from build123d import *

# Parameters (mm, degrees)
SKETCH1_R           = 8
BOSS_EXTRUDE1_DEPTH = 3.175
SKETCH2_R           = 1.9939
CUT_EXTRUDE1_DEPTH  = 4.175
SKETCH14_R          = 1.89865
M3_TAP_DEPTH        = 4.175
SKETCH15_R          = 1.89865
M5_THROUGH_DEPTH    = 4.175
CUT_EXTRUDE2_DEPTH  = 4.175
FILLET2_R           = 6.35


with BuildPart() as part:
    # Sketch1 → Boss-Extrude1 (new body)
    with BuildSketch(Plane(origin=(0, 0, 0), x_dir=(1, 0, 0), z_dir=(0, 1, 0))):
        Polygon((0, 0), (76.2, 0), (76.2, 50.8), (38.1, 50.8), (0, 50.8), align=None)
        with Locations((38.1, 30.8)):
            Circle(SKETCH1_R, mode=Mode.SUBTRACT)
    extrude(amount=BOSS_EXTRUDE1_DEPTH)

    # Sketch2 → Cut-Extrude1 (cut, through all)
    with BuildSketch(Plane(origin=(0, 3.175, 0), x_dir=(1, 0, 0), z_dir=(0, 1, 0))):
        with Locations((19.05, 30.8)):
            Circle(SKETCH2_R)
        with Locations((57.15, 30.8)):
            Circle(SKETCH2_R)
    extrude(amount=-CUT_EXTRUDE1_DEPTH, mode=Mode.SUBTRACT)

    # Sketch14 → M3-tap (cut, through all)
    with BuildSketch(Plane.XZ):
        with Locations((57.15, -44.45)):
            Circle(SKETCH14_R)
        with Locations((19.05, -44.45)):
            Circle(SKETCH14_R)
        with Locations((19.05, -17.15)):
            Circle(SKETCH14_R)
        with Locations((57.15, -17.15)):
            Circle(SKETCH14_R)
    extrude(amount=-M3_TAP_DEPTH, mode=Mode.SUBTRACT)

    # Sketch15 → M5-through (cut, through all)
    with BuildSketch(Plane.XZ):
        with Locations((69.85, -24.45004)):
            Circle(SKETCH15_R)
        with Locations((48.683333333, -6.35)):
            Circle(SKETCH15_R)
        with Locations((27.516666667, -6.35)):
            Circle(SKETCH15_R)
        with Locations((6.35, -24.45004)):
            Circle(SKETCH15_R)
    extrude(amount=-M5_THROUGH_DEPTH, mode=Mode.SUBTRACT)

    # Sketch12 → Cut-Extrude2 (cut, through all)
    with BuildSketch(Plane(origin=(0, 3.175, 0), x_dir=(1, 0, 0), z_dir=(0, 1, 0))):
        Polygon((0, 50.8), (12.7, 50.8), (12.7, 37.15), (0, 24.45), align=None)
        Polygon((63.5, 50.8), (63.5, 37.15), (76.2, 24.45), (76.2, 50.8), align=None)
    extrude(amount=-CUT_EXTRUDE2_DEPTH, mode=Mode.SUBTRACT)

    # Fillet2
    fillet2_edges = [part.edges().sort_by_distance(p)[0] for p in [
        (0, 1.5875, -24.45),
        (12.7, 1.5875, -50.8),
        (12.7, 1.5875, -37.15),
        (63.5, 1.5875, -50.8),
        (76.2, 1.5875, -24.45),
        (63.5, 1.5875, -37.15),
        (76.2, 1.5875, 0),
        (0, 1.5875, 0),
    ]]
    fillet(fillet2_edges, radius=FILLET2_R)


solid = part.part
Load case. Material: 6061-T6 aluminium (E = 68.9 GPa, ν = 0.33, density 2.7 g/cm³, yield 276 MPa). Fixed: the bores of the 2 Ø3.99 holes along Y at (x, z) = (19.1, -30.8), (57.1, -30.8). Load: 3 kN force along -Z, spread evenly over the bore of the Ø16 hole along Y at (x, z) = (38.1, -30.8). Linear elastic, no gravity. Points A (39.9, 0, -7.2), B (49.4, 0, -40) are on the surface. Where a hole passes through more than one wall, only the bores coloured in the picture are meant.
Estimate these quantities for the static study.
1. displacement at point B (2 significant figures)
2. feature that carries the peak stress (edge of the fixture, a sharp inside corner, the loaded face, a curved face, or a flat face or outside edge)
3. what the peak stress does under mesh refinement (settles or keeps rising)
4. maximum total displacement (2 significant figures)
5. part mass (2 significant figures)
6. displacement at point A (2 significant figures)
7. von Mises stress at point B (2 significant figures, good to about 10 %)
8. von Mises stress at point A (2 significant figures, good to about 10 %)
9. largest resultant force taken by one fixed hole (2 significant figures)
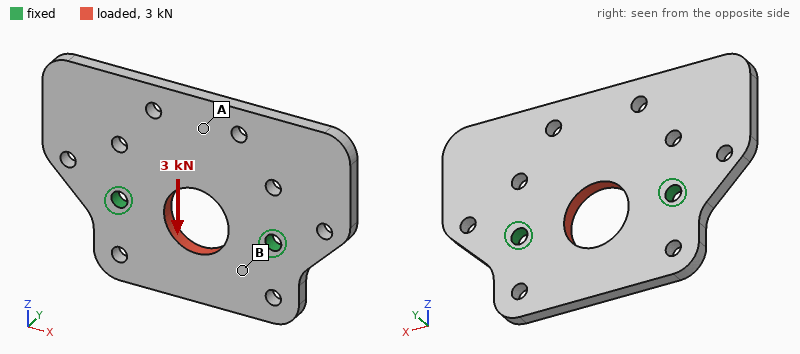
6.5 µm
edge of the fixture
keeps rising
12 µm
26 g
7.1 µm
22 MPa
8.6 MPa
1.5 kN
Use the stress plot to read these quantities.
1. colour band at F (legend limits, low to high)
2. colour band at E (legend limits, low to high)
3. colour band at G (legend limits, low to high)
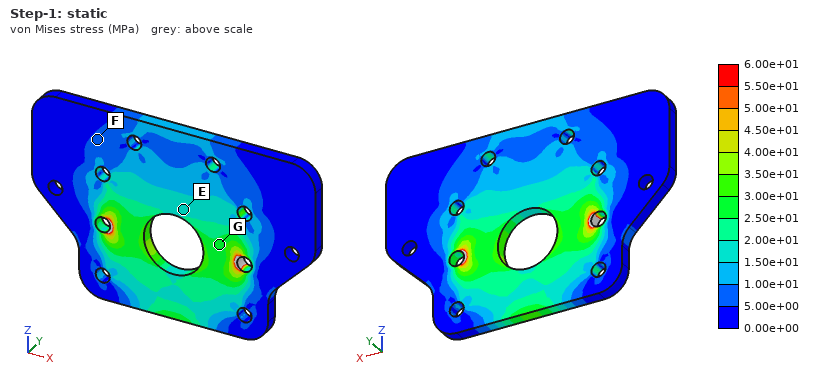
5.00e+00 to 1.00e+01 MPa
1.50e+01 to 2.00e+01 MPa
2.50e+01 to 3.00e+01 MPa
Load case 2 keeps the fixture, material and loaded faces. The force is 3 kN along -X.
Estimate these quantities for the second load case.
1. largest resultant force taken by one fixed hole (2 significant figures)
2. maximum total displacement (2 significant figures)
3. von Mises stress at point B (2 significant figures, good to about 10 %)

1.5 kN
8.3 µm
15 MPa
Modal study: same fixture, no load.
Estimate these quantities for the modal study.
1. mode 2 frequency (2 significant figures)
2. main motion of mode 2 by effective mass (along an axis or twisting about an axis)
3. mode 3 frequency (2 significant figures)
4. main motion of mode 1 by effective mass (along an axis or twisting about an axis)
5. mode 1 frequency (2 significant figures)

3000 Hz
twisting about Z
4600 Hz
along Y
2300 Hz
